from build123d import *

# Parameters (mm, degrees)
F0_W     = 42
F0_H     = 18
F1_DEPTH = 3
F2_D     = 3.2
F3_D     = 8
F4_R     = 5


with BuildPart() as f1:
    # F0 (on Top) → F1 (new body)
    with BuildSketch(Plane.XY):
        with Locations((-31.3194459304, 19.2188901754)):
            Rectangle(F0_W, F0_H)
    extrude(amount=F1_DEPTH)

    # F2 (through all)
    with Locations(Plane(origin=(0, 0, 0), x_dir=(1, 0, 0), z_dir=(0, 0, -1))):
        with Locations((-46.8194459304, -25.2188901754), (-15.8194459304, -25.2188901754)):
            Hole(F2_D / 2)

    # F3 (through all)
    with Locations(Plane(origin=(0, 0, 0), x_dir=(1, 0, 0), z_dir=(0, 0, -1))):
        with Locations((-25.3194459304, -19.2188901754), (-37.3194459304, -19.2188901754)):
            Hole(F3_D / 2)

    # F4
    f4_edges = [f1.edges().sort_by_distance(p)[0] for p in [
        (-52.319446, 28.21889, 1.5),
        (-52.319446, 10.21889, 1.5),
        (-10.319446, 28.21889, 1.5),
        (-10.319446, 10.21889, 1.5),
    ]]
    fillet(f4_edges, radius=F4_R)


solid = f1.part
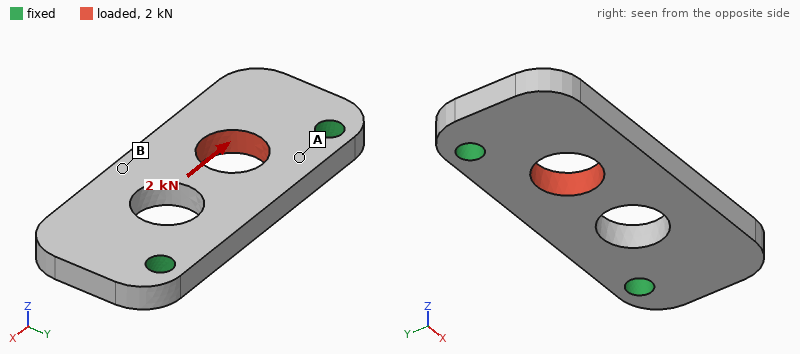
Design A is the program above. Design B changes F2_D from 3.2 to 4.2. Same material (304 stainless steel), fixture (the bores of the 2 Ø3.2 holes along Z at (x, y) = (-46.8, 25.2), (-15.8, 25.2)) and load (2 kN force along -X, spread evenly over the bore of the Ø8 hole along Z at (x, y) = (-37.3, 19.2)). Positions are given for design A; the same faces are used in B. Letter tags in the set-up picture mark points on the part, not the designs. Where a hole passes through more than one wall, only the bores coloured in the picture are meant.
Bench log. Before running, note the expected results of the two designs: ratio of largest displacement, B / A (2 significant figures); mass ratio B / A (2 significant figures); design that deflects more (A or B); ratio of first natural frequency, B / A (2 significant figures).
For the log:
0.91
0.98
A
1.1
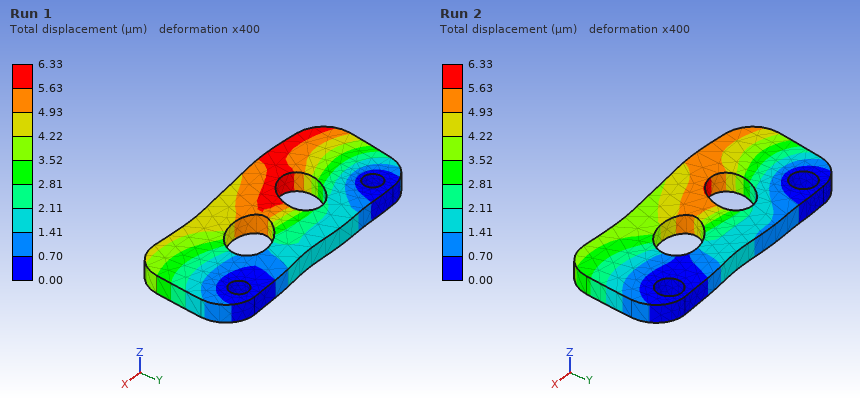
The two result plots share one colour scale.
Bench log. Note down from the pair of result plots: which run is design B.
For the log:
Run 2
